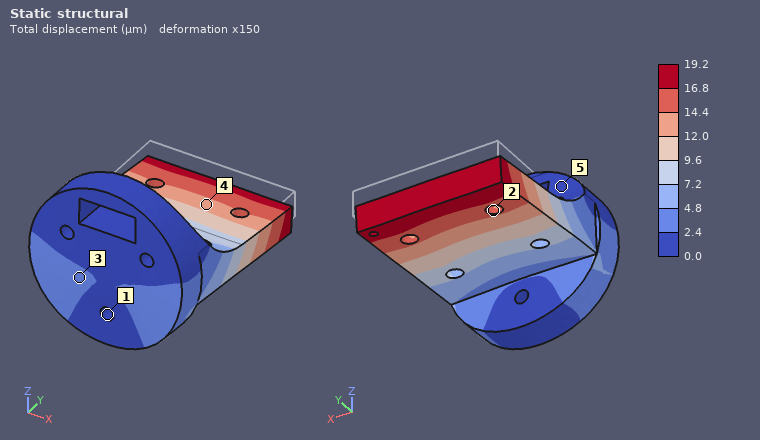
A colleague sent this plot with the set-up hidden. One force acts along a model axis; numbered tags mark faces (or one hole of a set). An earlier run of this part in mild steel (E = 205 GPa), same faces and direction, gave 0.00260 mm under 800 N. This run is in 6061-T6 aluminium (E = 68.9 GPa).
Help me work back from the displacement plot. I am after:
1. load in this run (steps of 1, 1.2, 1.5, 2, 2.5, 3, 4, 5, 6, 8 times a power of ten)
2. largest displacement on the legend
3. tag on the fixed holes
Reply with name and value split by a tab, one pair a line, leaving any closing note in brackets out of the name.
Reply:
load in this run	2 kN
largest displacement on the legend	19.2 µm
tag on the fixed holes	1
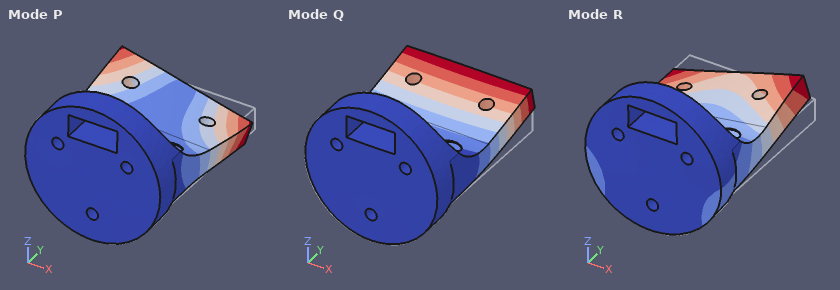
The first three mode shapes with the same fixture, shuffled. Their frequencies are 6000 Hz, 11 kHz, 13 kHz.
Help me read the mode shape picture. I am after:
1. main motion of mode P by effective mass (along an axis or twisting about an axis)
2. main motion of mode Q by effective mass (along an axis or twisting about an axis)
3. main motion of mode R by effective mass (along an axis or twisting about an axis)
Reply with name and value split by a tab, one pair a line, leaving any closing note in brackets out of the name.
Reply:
main motion of mode P by effective mass	along X
main motion of mode Q by effective mass	along Z
main motion of mode R by effective mass	along X
